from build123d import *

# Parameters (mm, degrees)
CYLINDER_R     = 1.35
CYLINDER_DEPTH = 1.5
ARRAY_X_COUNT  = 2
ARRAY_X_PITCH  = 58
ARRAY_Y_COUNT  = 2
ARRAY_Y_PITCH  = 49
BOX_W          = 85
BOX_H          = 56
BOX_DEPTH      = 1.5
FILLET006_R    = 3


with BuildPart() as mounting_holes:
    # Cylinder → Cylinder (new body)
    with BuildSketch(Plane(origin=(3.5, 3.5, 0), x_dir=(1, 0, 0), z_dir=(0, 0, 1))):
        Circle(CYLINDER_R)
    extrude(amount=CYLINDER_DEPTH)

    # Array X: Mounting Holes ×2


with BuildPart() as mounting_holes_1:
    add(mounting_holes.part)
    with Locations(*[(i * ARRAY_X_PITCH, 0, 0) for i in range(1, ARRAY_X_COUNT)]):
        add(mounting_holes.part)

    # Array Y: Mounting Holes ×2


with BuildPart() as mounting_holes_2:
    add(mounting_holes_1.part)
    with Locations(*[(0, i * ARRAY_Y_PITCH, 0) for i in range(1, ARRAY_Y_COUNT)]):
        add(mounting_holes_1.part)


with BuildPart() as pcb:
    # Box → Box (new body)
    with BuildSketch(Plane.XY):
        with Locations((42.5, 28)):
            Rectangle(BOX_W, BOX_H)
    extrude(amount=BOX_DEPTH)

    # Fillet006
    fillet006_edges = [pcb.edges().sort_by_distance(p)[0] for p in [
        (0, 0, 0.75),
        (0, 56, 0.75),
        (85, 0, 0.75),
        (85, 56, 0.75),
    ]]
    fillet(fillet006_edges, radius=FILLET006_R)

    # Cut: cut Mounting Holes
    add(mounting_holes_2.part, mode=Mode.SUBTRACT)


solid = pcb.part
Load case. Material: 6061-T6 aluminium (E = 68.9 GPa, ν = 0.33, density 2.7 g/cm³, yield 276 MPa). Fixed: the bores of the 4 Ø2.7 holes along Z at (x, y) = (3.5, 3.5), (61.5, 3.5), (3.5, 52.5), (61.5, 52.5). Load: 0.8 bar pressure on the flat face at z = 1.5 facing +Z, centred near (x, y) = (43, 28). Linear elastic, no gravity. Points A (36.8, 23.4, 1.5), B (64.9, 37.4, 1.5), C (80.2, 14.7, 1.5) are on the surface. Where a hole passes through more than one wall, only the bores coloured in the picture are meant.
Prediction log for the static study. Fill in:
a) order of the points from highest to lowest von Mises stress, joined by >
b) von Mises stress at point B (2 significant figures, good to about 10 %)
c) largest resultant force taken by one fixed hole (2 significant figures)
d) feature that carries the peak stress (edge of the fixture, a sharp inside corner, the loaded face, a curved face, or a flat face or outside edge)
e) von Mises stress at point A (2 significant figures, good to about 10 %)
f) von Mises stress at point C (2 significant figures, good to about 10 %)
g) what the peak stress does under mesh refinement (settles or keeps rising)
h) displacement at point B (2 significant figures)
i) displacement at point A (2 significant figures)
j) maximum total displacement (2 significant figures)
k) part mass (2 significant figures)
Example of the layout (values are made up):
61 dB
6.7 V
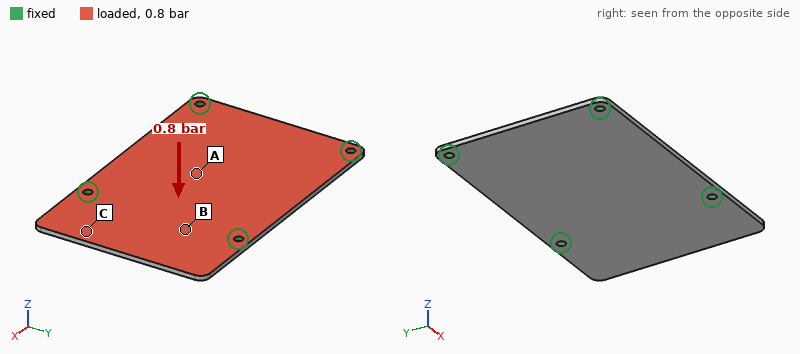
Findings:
B > A > C
40 MPa
120 N
edge of the fixture
28 MPa
12 MPa
keeps rising
0.099 mm
0.21 mm
0.25 mm
19 g
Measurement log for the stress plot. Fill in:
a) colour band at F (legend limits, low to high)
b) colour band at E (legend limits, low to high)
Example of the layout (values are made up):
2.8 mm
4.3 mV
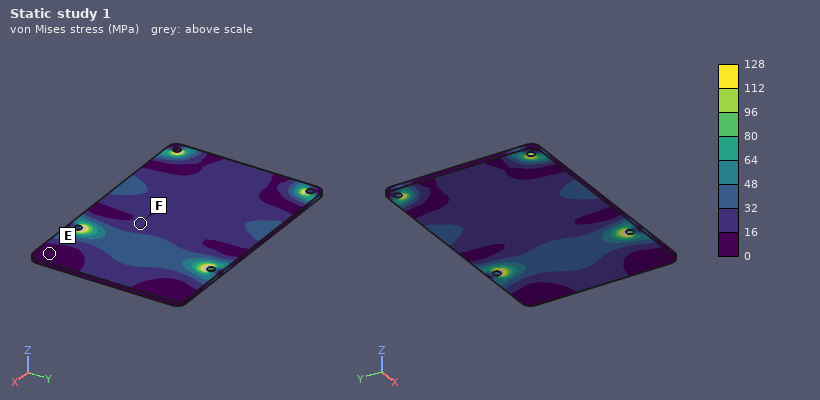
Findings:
16 to 32 MPa
0 to 16 MPa
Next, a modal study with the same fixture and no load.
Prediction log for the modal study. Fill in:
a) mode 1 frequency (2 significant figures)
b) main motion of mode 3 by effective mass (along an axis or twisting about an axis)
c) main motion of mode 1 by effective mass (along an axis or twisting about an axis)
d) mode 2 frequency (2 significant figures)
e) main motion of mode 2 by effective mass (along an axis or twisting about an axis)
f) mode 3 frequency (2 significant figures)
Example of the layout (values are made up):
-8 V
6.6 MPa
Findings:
1600 Hz
twisting about X
twisting about Y
1800 Hz
along Z
2800 Hz
